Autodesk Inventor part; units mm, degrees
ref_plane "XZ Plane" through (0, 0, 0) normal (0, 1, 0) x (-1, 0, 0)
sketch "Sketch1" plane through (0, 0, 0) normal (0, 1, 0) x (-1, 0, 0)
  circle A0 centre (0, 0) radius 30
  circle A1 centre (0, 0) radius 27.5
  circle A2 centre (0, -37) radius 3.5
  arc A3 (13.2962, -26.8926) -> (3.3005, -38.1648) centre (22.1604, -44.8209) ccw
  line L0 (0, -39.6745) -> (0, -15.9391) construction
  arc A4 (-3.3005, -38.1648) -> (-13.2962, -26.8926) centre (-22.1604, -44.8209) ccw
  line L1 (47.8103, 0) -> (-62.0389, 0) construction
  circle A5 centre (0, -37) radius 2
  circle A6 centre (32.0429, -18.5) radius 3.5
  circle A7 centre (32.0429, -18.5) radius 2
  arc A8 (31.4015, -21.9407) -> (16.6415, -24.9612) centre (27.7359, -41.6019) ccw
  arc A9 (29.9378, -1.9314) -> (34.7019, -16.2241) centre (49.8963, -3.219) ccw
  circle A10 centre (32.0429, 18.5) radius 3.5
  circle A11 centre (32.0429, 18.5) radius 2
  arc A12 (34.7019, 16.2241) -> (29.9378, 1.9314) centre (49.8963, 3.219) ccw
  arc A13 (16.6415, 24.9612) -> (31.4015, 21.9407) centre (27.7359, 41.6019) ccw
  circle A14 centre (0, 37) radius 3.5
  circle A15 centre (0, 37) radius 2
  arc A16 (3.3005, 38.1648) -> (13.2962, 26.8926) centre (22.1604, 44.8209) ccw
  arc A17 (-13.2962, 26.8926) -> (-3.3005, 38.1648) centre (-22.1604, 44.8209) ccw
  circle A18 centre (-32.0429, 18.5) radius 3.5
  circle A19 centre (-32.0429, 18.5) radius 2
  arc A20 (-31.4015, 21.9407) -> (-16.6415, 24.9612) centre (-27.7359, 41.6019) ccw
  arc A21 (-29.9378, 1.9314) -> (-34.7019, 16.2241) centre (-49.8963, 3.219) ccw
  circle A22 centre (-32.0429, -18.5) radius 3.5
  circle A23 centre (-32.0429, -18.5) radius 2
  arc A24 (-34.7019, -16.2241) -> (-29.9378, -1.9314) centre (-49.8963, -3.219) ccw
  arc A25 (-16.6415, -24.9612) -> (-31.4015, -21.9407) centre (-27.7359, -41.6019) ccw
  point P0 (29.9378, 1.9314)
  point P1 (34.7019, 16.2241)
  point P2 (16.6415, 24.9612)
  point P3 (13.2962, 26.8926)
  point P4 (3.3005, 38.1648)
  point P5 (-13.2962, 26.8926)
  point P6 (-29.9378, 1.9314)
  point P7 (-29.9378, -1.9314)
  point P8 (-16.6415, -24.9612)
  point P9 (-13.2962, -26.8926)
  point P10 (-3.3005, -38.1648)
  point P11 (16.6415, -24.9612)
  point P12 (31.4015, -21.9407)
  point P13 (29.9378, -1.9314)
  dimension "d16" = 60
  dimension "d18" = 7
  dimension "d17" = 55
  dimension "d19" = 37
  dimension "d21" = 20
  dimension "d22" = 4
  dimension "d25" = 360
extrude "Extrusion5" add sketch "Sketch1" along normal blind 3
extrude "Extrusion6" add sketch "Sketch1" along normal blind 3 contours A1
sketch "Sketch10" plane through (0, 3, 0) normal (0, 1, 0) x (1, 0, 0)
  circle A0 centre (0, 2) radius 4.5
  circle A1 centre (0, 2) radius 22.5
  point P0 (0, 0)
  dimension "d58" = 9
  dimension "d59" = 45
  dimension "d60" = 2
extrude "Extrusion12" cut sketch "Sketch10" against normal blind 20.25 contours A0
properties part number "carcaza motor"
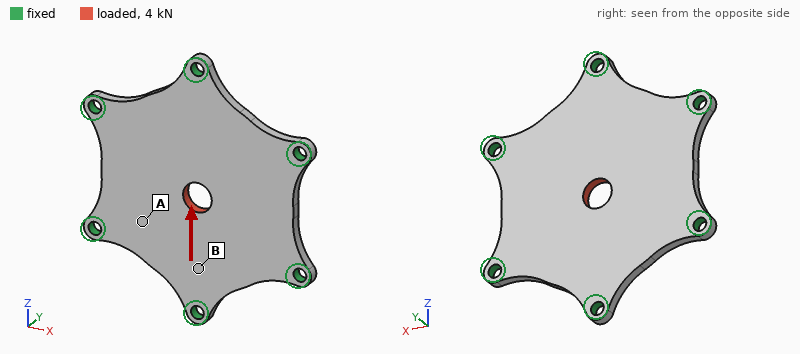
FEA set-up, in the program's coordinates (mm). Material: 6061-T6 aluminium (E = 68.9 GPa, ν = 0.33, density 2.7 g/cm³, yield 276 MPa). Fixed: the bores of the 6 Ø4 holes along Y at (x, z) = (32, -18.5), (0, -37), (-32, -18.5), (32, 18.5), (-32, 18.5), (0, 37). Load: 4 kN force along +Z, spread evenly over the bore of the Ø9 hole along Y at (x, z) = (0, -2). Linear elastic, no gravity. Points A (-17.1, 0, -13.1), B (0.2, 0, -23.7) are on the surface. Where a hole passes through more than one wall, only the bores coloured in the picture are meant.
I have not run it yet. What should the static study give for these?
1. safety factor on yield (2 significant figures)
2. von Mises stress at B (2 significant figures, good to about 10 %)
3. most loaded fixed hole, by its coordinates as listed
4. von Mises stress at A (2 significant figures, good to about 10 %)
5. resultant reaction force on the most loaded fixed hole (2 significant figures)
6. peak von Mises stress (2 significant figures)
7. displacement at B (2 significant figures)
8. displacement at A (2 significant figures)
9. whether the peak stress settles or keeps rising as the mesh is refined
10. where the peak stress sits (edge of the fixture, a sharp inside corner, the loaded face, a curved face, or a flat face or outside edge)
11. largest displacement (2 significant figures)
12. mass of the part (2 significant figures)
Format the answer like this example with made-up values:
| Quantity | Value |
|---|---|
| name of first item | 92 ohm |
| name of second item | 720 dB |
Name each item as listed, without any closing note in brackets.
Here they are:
| Quantity | Value |
|---|---|
| safety factor on yield | 3.4 |
| von Mises stress at B | 32 MPa |
| most loaded fixed hole, by its coordinates as listed | (0, -37) |
| von Mises stress at A | 13 MPa |
| resultant reaction force on the most loaded fixed hole | 1.2 kN |
| peak von Mises stress | 82 MPa |
| displacement at B | 6.4 µm |
| displacement at A | 6.2 µm |
| whether the peak stress settles or keeps rising as the mesh is refined | settles |
| where the peak stress sits | the loaded face |
| largest displacement | 15 µm |
| mass of the part | 27 g |
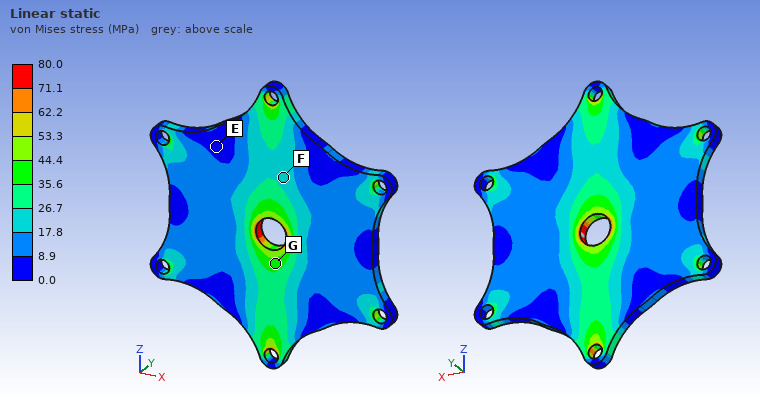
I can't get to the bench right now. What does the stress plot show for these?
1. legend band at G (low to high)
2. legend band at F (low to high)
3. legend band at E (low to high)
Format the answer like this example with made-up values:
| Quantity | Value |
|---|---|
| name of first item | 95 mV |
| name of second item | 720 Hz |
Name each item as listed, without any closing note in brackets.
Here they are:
| Quantity | Value |
|---|---|
| legend band at G | 35.6 to 44.4 MPa |
| legend band at F | 17.8 to 26.7 MPa |
| legend band at E | 0.0 to 8.9 MPa |
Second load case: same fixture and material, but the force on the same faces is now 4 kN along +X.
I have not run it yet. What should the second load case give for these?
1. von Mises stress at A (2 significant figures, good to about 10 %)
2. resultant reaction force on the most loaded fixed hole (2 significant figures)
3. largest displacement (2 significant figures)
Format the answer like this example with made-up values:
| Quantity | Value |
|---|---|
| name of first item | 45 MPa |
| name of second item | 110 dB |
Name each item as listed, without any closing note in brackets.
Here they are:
| Quantity | Value |
|---|---|
| von Mises stress at A | 26 MPa |
| resultant reaction force on the most loaded fixed hole | 1.0 kN |
| largest displacement | 15 µm |
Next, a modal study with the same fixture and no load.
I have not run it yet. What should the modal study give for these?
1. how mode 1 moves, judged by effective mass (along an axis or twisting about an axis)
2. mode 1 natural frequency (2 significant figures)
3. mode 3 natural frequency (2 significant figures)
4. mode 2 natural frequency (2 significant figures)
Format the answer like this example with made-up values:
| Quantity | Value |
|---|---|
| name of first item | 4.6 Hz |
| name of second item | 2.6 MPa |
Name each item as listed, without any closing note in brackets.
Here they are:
| Quantity | Value |
|---|---|
| how mode 1 moves, judged by effective mass | along Y |
| mode 1 natural frequency | 4200 Hz |
| mode 3 natural frequency | 8700 Hz |
| mode 2 natural frequency | 8700 Hz |
